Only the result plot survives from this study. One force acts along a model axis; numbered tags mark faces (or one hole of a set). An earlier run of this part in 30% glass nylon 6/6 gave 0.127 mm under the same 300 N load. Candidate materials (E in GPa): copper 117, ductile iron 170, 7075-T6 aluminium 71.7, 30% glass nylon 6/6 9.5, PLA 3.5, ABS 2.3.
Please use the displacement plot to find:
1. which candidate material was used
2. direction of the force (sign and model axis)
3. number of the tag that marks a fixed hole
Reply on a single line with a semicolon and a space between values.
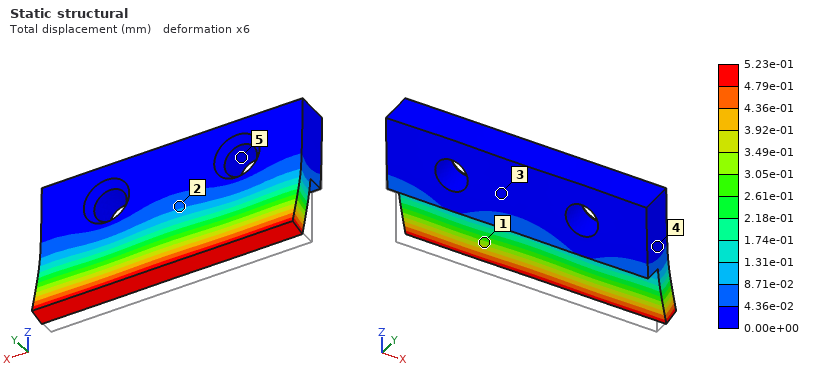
ABS; +Y; 5
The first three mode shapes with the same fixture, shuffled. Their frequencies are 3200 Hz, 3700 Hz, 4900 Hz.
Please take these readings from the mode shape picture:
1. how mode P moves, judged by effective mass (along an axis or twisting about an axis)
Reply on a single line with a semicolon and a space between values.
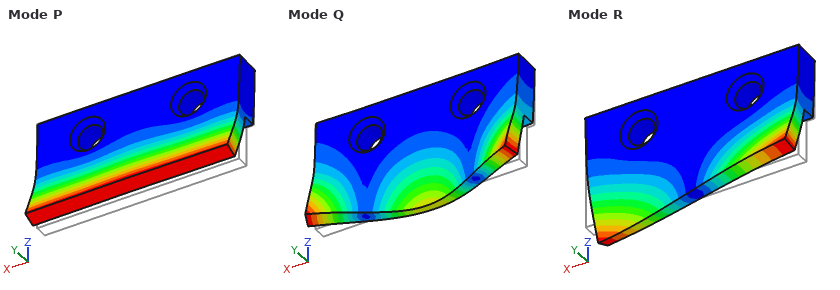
along Y
